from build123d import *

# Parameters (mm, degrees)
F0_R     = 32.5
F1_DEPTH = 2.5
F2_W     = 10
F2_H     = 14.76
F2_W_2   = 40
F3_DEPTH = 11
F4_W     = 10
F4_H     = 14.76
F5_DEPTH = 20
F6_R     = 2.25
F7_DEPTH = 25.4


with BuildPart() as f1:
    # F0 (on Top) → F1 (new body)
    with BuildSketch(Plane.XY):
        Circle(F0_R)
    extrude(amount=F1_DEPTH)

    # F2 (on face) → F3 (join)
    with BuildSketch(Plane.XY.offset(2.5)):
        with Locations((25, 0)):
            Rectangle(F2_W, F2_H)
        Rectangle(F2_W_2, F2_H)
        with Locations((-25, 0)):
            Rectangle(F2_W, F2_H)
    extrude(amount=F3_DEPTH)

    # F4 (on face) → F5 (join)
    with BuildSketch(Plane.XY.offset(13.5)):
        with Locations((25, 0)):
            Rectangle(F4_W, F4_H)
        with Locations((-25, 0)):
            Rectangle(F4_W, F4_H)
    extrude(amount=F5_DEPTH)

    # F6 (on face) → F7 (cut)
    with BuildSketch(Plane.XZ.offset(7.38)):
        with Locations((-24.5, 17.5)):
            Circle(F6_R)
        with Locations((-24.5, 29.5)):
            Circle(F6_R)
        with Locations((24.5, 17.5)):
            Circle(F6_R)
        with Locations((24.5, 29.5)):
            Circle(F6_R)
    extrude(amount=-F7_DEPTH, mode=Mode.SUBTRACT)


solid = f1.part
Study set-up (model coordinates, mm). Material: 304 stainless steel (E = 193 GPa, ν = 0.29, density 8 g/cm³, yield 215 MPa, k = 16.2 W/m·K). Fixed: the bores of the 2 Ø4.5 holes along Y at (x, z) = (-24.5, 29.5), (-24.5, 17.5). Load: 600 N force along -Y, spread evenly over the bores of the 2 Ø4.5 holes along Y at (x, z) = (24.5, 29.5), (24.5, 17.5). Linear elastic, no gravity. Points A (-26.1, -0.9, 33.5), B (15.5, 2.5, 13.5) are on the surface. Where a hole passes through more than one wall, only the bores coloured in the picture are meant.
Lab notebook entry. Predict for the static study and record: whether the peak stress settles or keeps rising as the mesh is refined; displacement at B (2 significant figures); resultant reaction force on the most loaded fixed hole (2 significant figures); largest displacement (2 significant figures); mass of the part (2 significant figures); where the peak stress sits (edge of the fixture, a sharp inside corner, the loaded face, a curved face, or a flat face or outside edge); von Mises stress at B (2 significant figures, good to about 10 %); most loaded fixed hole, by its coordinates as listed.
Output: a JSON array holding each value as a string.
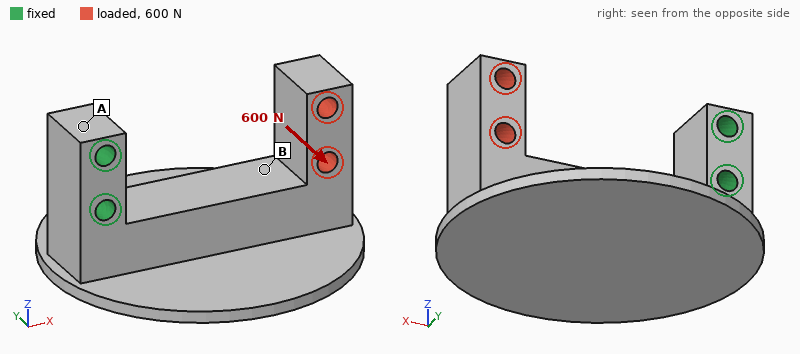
["keeps rising", "47 µm", "600 N", "94 µm", "180 g", "edge of the fixture", "35 MPa", "(-24.5, 17.5)"]
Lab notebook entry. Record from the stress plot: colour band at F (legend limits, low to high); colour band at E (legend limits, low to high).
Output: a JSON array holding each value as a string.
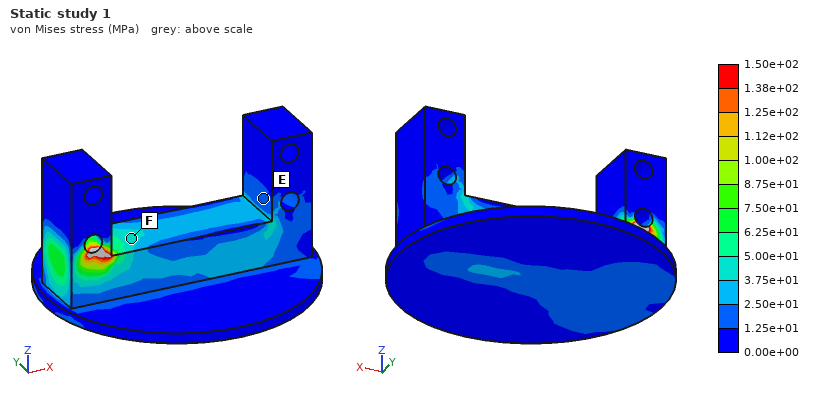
["3.75e+01 to 5.00e+01 MPa", "1.25e+01 to 2.50e+01 MPa"]
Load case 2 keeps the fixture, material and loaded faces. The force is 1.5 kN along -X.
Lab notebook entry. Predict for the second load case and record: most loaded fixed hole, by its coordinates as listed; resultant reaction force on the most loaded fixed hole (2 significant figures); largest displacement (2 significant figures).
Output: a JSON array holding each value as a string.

["(-24.5, 17.5)", "1.3 kN", "0.11 mm"]
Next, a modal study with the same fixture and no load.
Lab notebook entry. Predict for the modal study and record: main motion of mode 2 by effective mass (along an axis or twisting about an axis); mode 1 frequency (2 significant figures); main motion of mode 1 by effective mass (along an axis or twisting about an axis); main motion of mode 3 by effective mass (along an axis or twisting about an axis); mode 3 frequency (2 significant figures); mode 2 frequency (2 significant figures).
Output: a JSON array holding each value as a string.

["along Y", "1500 Hz", "along Z", "twisting about X", "3000 Hz", "1900 Hz"]
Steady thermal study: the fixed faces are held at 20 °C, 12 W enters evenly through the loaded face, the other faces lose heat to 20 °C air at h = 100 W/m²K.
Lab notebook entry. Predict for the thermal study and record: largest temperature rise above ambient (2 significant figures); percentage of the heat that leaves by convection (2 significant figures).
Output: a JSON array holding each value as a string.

["66 K", "96 %"]
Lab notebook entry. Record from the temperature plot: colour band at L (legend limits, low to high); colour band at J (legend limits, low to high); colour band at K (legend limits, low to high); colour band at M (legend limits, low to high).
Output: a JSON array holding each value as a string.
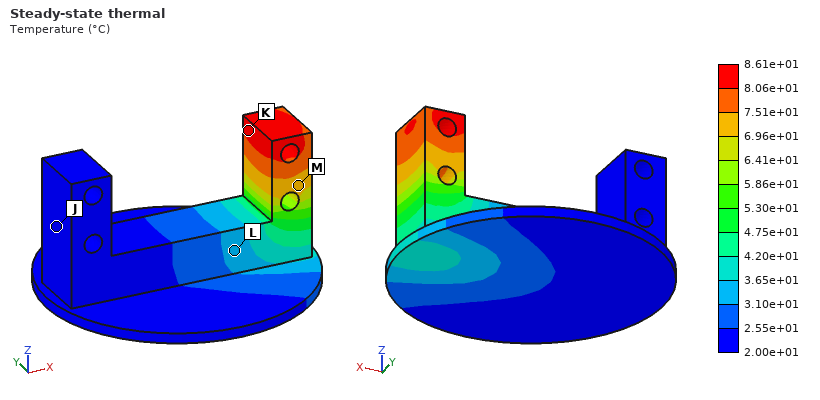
["3.10e+01 to 3.65e+01 °C", "2.00e+01 to 2.55e+01 °C", "8.06e+01 to 8.61e+01 °C", "6.96e+01 to 7.51e+01 °C"]
